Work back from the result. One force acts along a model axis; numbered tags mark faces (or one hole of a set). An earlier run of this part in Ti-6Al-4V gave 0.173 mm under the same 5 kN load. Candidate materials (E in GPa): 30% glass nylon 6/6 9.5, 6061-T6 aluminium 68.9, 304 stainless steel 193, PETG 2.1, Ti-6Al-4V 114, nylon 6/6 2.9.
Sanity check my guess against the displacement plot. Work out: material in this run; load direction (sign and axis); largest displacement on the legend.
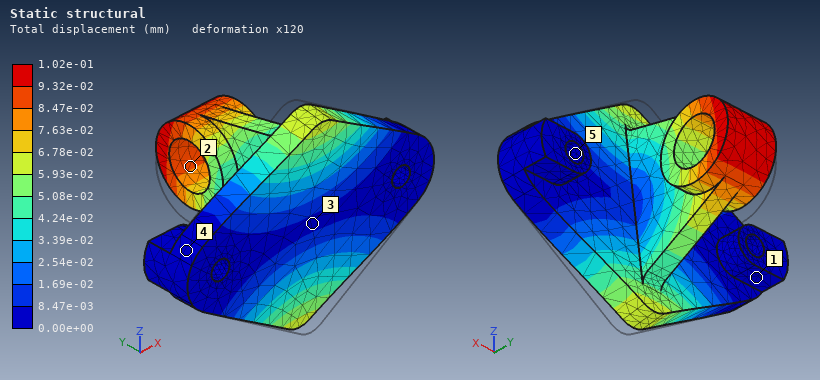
304 stainless steel
+Z
1.02e-01 mm
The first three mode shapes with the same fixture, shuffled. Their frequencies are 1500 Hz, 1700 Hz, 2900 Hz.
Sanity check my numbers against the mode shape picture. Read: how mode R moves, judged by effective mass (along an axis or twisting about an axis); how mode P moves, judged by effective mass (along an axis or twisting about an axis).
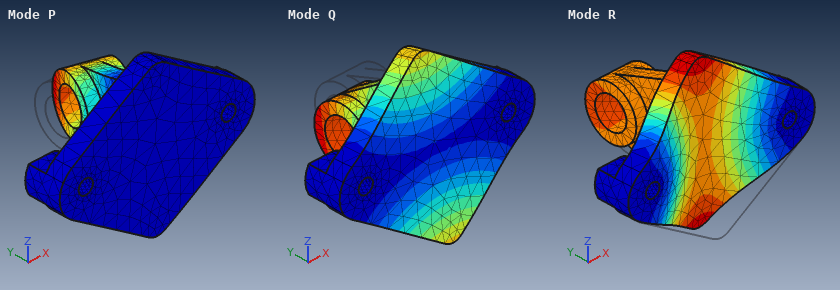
along Y
along X
